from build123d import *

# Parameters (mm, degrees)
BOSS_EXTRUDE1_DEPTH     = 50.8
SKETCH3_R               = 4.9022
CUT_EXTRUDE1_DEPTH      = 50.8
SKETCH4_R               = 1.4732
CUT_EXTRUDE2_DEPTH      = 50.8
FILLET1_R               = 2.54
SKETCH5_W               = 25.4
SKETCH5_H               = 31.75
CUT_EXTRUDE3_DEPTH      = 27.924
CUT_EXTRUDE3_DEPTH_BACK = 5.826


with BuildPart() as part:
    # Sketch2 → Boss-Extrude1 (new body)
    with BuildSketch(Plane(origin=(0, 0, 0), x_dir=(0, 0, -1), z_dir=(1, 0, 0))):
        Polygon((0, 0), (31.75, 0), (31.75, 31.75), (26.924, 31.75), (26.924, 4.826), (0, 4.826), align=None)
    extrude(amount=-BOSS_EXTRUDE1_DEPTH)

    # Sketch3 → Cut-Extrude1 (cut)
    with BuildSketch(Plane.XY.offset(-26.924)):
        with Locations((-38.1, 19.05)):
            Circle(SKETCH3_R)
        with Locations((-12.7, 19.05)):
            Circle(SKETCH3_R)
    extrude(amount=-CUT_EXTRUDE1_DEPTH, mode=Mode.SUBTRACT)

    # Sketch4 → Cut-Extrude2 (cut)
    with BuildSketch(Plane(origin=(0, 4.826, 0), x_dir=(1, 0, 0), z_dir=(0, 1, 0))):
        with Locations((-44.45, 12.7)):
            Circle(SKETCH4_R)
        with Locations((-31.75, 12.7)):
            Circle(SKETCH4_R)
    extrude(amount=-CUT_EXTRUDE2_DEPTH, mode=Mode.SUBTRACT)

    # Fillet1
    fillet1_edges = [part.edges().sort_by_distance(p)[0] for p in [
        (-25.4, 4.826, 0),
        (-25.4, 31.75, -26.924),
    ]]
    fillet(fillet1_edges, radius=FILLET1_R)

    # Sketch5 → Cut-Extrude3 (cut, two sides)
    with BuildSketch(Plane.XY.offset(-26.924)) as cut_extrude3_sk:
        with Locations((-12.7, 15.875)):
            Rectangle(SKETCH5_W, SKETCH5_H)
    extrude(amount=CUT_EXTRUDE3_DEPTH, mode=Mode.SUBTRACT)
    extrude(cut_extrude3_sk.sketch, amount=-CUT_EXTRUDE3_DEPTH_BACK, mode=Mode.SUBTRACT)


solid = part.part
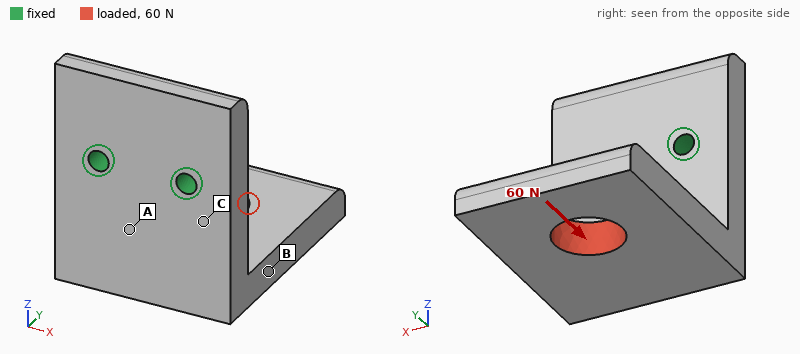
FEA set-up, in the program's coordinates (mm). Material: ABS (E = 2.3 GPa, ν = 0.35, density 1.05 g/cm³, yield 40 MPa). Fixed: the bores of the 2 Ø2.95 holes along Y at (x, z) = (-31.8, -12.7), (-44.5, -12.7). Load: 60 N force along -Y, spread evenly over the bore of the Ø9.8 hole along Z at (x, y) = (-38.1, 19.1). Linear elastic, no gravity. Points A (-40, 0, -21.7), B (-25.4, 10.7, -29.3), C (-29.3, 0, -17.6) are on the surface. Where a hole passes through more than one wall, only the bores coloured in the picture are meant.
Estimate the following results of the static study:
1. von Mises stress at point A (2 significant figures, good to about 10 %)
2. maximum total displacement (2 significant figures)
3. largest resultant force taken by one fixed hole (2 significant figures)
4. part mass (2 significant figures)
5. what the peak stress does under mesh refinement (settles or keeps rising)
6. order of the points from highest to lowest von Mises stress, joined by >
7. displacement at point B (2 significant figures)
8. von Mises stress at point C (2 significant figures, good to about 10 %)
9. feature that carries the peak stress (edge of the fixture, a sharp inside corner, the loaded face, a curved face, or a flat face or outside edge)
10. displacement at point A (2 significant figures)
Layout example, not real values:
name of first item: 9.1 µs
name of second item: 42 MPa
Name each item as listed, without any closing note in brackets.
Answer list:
von Mises stress at point A: 4.1 MPa
maximum total displacement: 0.49 mm
largest resultant force taken by one fixed hole: 30 N
part mass: 7.0 g
what the peak stress does under mesh refinement: keeps rising
order of the points from highest to lowest von Mises stress, joined by >: C > A > B
displacement at point B: 0.22 mm
von Mises stress at point C: 6.7 MPa
feature that carries the peak stress: edge of the fixture
displacement at point A: 0.075 mm
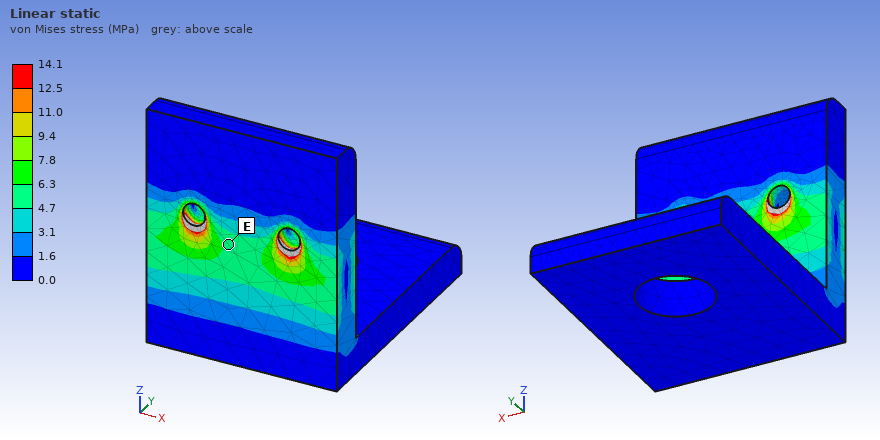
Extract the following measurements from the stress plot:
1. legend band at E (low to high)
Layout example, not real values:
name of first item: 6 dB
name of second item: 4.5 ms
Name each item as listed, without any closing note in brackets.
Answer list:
legend band at E: 4.7 to 6.3 MPa
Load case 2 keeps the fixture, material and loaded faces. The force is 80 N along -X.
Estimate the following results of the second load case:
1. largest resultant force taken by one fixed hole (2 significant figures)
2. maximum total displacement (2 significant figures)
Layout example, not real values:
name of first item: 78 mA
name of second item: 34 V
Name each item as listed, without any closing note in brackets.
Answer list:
largest resultant force taken by one fixed hole: 120 N
maximum total displacement: 0.58 mm
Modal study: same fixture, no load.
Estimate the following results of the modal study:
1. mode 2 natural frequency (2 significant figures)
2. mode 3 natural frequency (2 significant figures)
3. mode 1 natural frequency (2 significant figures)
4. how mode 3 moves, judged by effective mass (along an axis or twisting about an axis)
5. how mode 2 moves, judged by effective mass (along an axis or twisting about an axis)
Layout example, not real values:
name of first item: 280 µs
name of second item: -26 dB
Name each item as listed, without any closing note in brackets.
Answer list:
mode 2 natural frequency: 1300 Hz
mode 3 natural frequency: 2200 Hz
mode 1 natural frequency: 750 Hz
how mode 3 moves, judged by effective mass: along Y
how mode 2 moves, judged by effective mass: along X
